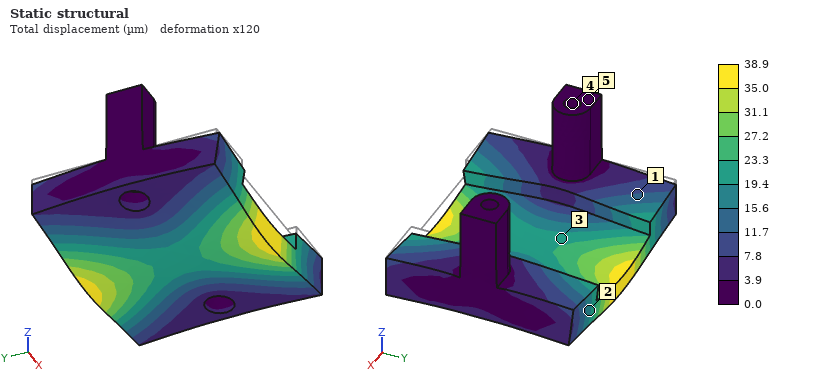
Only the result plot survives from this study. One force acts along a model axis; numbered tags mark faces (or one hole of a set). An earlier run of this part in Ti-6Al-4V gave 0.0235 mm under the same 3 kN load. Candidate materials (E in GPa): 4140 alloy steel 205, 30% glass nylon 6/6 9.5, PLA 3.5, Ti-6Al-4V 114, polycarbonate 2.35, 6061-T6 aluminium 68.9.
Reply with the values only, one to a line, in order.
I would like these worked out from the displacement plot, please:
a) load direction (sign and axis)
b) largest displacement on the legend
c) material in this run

-Z
38.9 µm
6061-T6 aluminium
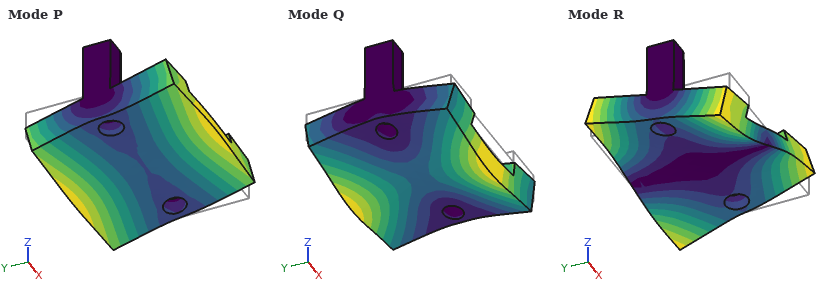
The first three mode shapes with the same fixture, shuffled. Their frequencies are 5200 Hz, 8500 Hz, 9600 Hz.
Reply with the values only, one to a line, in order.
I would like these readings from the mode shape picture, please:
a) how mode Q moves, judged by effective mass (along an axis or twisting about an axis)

along Z
